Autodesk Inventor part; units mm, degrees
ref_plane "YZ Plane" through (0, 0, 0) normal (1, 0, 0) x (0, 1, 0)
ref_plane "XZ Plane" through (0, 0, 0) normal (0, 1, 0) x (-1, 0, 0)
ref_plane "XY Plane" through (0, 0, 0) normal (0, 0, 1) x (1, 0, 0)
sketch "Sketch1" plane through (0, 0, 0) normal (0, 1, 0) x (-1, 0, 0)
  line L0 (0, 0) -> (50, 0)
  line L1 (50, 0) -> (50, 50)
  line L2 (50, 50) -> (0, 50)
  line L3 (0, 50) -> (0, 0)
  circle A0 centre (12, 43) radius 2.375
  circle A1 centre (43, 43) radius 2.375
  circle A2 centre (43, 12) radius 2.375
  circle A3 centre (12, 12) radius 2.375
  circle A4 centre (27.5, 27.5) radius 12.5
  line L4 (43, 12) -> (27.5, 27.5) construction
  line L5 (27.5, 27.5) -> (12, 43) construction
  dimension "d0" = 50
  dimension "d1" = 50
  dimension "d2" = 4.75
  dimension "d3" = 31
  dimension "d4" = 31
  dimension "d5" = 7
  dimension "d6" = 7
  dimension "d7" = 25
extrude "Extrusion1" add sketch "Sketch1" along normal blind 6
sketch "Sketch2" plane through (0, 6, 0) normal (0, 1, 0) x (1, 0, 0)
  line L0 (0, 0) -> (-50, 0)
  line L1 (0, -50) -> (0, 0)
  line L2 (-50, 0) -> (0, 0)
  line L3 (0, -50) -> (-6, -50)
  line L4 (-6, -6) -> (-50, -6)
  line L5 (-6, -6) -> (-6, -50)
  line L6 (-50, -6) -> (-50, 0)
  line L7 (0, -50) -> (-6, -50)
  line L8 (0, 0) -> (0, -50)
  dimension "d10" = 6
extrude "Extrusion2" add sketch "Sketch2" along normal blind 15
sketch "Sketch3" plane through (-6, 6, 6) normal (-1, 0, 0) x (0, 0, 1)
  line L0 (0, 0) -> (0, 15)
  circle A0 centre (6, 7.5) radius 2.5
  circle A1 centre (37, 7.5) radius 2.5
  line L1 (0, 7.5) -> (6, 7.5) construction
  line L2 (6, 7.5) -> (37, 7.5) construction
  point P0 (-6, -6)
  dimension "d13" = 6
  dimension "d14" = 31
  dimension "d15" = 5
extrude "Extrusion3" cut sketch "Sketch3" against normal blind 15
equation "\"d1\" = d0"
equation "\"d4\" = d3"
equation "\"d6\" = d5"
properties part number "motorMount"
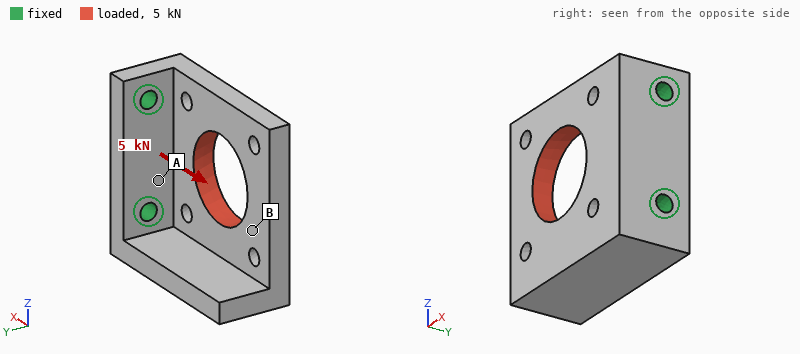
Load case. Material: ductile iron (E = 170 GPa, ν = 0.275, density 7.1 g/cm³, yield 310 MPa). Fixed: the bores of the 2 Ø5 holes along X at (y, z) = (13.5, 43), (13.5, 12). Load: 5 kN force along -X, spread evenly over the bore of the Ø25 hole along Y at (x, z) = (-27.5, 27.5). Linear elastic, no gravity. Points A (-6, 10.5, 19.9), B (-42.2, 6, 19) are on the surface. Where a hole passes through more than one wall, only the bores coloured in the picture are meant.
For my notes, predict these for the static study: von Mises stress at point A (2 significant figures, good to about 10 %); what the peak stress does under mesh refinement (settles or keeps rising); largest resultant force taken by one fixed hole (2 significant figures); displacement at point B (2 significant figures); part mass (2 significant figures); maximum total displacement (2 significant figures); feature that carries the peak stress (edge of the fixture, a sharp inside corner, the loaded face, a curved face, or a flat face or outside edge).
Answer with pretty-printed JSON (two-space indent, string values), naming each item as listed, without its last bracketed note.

{
  "von Mises stress at point A": "54 MPa",
  "what the peak stress does under mesh refinement": "keeps rising",
  "largest resultant force taken by one fixed hole": "2.5 kN",
  "displacement at point B": "64 µm",
  "part mass": "140 g",
  "maximum total displacement": "89 µm",
  "feature that carries the peak stress": "edge of the fixture"
}
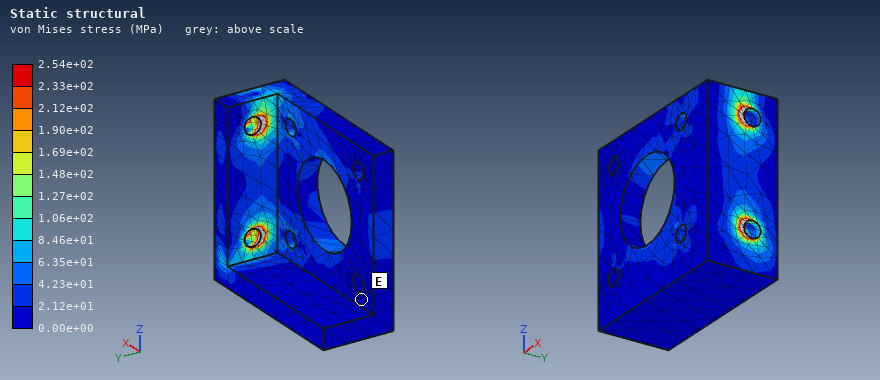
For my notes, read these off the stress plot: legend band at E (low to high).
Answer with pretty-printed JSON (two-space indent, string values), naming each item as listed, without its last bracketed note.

{
  "legend band at E": "0.00e+00 to 2.12e+01 MPa"
}
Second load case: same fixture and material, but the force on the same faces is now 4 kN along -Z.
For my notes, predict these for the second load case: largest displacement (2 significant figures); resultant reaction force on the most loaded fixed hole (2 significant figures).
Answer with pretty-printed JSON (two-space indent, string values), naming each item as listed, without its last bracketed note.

{
  "largest displacement": "88 µm",
  "resultant reaction force on the most loaded fixed hole": "3.5 kN"
}
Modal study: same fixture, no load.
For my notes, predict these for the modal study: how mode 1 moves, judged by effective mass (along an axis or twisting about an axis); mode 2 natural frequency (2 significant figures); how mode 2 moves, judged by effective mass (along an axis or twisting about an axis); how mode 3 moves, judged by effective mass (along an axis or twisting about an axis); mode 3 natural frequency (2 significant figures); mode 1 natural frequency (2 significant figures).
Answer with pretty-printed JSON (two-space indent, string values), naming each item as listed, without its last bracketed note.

{
  "how mode 1 moves, judged by effective mass": "along Y",
  "mode 2 natural frequency": "3400 Hz",
  "how mode 2 moves, judged by effective mass": "along Z",
  "how mode 3 moves, judged by effective mass": "along Z",
  "mode 3 natural frequency": "5400 Hz",
  "mode 1 natural frequency": "2100 Hz"
}
